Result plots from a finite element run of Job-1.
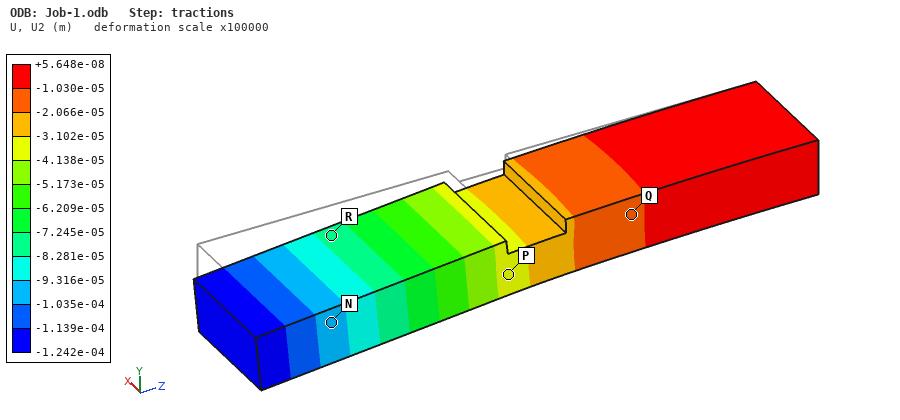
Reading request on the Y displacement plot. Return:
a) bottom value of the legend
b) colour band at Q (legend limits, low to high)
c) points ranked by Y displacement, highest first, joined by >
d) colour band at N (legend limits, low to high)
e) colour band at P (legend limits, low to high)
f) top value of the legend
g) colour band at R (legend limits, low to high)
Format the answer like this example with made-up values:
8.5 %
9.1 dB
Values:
-1.242e-04 m
-2.066e-05 to -1.030e-05 m
Q > P > R > N
-1.035e-04 to -9.316e-05 m
-4.138e-05 to -3.102e-05 m
+5.648e-08 m
-8.281e-05 to -7.245e-05 m
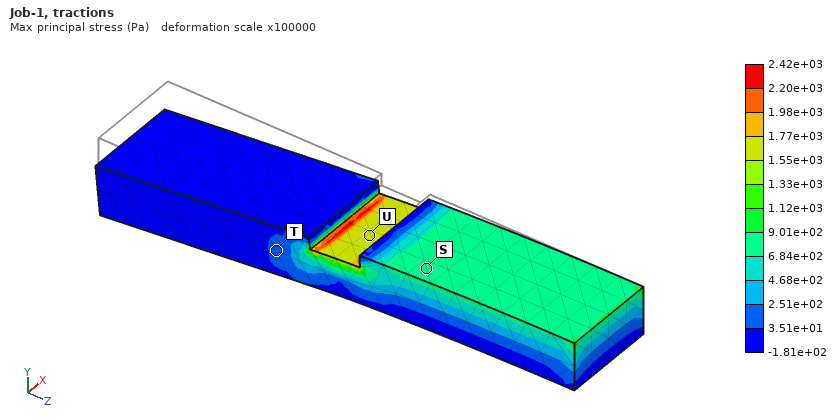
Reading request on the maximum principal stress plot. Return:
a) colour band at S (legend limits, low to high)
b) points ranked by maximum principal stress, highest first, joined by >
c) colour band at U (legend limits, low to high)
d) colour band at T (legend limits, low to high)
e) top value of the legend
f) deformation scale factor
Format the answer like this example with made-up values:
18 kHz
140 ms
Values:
6.84e+02 to 9.01e+02 Pa
U > S > T
1.55e+03 to 1.77e+03 Pa
3.51e+01 to 2.51e+02 Pa
2.42e+03 Pa
100000
